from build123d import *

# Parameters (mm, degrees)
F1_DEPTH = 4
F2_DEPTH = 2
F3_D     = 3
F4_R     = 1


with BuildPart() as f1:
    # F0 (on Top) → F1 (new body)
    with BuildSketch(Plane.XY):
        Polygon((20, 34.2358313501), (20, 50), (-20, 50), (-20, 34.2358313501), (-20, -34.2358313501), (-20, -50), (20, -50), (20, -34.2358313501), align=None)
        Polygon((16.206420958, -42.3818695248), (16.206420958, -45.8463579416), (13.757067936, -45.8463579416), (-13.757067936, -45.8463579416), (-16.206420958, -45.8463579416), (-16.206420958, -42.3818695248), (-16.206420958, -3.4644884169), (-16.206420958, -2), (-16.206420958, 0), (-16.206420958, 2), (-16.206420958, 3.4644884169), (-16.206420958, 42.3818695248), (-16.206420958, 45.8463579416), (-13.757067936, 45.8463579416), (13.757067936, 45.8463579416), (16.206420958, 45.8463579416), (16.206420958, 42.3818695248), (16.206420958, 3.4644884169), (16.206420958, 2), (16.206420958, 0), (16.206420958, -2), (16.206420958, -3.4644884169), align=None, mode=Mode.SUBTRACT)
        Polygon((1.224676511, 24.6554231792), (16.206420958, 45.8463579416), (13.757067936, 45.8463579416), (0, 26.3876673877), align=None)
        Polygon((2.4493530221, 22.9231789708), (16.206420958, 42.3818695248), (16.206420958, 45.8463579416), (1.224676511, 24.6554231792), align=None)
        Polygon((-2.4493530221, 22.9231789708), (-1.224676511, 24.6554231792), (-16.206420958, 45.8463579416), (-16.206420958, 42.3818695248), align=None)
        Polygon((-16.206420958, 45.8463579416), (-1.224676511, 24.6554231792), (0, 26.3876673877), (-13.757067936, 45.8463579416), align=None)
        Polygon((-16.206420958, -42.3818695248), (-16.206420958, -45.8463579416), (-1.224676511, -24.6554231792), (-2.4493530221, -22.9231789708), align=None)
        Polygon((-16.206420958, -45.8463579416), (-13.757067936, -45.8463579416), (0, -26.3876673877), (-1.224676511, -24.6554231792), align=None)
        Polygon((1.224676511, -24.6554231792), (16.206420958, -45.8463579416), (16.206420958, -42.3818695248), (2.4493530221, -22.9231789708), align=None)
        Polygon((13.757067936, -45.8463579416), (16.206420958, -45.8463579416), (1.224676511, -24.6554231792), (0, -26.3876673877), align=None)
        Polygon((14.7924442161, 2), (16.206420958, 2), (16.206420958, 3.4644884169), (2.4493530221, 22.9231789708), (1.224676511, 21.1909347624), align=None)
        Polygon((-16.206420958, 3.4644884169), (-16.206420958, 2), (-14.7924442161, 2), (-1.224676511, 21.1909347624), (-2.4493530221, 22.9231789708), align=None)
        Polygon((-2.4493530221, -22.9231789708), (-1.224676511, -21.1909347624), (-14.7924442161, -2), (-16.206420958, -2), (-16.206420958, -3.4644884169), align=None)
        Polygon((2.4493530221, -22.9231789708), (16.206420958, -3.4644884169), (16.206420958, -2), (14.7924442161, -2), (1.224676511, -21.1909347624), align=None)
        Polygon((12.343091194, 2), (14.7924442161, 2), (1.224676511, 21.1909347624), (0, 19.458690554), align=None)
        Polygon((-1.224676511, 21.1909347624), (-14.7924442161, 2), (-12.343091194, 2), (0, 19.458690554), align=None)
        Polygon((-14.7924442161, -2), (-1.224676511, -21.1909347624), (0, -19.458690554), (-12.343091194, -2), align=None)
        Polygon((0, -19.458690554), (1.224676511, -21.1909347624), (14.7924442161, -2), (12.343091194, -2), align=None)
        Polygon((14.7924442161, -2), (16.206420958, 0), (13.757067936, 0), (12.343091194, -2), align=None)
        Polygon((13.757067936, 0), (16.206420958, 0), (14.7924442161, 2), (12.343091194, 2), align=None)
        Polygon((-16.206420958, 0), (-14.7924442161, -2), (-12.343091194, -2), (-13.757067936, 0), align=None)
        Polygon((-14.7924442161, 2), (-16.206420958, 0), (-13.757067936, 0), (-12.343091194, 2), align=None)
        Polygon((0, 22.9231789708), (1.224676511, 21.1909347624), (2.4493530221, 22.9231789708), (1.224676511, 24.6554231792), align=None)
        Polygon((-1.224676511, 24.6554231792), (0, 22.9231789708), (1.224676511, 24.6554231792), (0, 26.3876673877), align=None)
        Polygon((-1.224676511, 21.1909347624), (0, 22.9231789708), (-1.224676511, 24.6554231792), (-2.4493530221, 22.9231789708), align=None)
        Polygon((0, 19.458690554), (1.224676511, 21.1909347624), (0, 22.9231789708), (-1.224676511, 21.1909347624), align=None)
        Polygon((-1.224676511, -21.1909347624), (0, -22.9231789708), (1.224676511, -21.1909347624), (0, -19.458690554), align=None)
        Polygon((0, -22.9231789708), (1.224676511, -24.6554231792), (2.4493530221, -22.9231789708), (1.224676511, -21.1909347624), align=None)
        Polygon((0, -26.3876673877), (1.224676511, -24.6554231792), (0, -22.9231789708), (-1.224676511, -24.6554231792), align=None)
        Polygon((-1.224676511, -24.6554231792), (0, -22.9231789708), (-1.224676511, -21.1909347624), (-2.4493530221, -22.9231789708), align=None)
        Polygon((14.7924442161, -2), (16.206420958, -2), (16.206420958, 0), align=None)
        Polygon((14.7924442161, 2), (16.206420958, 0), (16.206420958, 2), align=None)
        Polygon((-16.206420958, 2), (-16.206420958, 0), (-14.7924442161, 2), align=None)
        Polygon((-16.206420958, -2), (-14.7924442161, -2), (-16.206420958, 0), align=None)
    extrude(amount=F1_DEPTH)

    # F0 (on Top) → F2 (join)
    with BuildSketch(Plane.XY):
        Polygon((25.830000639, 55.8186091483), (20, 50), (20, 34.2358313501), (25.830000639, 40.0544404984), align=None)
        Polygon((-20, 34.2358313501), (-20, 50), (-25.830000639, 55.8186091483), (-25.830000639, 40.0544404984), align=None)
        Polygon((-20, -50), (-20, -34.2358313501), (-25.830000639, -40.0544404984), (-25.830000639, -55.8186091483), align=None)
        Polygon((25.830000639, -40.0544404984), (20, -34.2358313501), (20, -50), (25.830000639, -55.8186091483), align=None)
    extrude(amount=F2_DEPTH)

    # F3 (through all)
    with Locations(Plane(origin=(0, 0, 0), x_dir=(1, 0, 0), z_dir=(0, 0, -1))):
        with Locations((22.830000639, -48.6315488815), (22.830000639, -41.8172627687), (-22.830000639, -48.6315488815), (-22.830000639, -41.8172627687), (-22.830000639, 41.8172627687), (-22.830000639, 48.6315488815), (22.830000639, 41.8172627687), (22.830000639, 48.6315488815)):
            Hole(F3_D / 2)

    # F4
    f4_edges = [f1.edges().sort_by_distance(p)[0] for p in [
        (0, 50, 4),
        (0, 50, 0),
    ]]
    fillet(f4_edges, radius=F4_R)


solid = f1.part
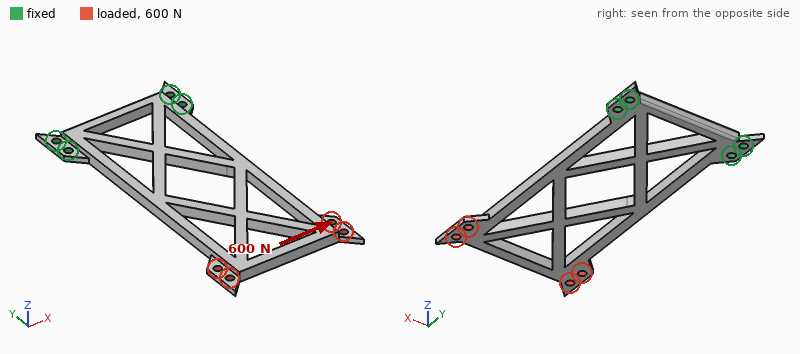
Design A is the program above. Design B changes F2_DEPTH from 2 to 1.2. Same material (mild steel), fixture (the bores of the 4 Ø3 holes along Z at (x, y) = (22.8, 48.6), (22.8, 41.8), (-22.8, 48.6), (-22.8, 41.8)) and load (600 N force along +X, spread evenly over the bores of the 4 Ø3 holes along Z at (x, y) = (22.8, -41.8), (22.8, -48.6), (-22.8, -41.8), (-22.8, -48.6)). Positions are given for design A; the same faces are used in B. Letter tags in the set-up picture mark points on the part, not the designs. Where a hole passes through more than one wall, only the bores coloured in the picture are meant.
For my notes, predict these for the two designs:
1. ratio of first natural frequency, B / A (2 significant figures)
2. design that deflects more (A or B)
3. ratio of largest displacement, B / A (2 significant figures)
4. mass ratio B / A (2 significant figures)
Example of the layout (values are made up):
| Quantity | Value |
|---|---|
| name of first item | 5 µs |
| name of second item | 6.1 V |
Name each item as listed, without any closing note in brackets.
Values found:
| Quantity | Value |
|---|---|
| ratio of first natural frequency, B / A | 0.97 |
| design that deflects more | B |
| ratio of largest displacement, B / A | 1.3 |
| mass ratio B / A | 0.97 |
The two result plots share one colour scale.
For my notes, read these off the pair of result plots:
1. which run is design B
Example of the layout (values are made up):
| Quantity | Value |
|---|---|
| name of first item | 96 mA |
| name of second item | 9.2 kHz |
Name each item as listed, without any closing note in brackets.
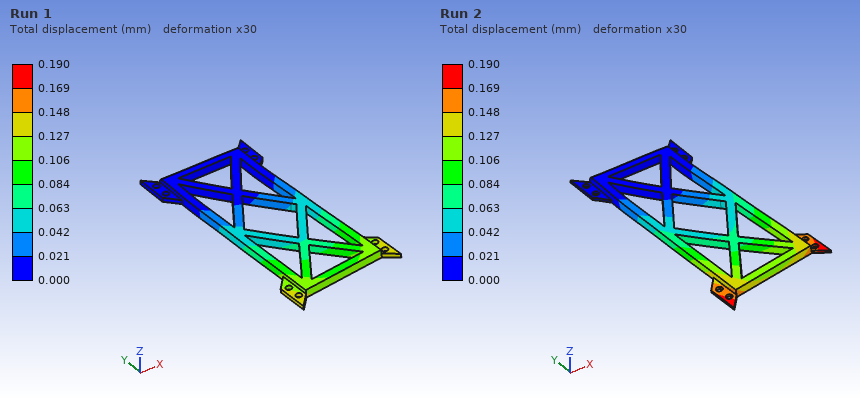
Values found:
| Quantity | Value |
|---|---|
| which run is design B | Run 2 |
